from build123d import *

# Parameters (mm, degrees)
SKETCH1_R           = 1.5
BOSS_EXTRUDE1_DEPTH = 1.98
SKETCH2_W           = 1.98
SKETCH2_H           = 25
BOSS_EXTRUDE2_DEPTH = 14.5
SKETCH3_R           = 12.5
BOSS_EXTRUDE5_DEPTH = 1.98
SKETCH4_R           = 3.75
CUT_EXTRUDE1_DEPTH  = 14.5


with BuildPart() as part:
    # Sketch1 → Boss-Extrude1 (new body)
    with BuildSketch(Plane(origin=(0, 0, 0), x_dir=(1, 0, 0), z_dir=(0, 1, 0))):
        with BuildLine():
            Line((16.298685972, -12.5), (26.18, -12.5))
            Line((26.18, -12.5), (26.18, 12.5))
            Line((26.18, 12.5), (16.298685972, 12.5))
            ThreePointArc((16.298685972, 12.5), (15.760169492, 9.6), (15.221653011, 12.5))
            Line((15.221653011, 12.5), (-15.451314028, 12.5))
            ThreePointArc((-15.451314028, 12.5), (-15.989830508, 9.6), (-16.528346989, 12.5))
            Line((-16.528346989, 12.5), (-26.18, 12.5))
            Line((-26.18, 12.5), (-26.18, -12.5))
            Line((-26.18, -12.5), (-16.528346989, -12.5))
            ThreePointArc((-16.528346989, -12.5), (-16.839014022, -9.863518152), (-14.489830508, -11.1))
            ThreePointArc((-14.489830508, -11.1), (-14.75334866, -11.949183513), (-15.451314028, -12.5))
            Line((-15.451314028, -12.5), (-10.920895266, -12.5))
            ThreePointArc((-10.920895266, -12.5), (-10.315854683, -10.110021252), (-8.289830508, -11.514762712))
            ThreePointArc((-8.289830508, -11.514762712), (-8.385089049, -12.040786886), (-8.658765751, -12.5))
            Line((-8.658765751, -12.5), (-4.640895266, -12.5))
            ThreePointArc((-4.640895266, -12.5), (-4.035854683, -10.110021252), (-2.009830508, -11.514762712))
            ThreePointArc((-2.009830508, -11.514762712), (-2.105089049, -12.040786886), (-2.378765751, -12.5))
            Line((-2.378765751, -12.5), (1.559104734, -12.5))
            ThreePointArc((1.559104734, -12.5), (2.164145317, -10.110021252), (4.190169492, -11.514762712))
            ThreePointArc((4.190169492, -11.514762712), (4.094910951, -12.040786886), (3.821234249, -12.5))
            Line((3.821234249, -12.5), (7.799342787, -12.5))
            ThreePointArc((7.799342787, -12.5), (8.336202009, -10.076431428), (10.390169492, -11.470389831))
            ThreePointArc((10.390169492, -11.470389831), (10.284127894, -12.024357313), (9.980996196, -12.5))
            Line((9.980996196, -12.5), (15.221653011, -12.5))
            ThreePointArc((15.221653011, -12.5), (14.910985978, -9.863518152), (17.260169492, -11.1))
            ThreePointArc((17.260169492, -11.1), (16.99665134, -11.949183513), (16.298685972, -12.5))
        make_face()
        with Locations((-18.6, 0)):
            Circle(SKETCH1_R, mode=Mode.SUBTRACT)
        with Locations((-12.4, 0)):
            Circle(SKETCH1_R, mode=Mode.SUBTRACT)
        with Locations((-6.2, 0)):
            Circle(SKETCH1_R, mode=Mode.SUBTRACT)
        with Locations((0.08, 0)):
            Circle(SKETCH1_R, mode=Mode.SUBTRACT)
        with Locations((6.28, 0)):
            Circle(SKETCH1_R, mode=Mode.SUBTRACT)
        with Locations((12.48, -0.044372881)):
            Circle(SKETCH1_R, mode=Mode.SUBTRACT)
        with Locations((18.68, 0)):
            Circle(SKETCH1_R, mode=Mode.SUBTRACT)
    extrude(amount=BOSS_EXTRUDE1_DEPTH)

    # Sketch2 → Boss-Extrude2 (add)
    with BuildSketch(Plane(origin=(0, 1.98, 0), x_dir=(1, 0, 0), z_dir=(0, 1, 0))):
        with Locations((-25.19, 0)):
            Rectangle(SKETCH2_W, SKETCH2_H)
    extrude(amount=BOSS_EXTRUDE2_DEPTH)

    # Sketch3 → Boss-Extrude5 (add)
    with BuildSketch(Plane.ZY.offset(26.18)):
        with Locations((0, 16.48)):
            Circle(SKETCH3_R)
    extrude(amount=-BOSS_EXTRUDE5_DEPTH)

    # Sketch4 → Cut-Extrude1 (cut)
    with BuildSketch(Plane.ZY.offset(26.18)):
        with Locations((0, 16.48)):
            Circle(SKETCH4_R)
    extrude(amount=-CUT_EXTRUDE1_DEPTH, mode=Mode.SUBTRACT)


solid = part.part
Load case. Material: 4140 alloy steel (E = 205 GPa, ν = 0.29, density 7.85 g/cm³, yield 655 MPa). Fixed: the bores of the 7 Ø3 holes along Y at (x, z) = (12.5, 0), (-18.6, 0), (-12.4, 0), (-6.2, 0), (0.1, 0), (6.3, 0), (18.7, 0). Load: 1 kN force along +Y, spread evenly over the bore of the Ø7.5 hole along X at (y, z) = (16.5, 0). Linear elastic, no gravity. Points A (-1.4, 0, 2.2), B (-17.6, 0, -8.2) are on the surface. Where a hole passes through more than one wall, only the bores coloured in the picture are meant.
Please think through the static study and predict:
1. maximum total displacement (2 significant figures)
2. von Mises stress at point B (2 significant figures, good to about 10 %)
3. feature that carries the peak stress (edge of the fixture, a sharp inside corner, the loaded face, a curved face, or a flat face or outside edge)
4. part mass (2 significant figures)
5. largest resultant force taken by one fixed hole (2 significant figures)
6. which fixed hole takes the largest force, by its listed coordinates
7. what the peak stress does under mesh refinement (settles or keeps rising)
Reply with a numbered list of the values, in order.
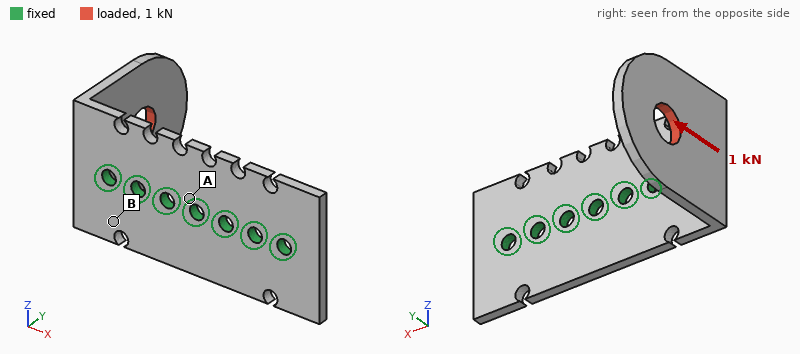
1. 0.22 mm
2. 150 MPa
3. edge of the fixture
4. 28 g
5. 1.3 kN
6. (-18.6, 0)
7. keeps rising
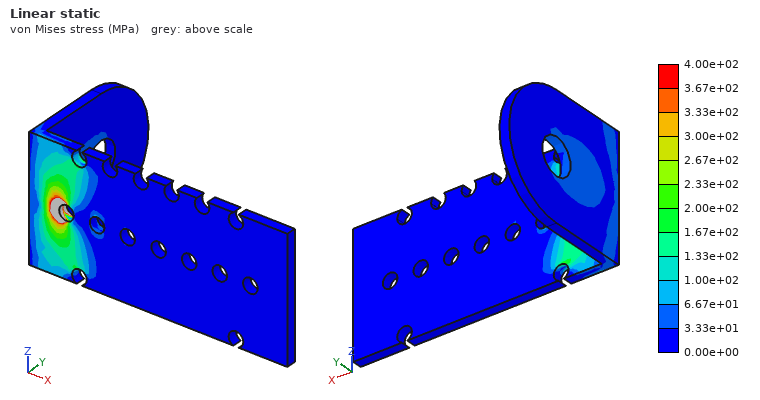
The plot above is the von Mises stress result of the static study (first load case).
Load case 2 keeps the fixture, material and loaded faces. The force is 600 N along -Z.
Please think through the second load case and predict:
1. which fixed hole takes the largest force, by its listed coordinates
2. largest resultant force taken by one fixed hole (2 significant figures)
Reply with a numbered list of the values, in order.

1. (-18.6, 0)
2. 720 N
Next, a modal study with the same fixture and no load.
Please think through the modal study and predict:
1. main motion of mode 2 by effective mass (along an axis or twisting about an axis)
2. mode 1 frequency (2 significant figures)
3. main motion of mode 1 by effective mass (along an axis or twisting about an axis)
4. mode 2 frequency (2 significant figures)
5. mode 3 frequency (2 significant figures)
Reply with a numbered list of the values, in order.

1. along Z
2. 1800 Hz
3. along X
4. 2800 Hz
5. 6300 Hz
